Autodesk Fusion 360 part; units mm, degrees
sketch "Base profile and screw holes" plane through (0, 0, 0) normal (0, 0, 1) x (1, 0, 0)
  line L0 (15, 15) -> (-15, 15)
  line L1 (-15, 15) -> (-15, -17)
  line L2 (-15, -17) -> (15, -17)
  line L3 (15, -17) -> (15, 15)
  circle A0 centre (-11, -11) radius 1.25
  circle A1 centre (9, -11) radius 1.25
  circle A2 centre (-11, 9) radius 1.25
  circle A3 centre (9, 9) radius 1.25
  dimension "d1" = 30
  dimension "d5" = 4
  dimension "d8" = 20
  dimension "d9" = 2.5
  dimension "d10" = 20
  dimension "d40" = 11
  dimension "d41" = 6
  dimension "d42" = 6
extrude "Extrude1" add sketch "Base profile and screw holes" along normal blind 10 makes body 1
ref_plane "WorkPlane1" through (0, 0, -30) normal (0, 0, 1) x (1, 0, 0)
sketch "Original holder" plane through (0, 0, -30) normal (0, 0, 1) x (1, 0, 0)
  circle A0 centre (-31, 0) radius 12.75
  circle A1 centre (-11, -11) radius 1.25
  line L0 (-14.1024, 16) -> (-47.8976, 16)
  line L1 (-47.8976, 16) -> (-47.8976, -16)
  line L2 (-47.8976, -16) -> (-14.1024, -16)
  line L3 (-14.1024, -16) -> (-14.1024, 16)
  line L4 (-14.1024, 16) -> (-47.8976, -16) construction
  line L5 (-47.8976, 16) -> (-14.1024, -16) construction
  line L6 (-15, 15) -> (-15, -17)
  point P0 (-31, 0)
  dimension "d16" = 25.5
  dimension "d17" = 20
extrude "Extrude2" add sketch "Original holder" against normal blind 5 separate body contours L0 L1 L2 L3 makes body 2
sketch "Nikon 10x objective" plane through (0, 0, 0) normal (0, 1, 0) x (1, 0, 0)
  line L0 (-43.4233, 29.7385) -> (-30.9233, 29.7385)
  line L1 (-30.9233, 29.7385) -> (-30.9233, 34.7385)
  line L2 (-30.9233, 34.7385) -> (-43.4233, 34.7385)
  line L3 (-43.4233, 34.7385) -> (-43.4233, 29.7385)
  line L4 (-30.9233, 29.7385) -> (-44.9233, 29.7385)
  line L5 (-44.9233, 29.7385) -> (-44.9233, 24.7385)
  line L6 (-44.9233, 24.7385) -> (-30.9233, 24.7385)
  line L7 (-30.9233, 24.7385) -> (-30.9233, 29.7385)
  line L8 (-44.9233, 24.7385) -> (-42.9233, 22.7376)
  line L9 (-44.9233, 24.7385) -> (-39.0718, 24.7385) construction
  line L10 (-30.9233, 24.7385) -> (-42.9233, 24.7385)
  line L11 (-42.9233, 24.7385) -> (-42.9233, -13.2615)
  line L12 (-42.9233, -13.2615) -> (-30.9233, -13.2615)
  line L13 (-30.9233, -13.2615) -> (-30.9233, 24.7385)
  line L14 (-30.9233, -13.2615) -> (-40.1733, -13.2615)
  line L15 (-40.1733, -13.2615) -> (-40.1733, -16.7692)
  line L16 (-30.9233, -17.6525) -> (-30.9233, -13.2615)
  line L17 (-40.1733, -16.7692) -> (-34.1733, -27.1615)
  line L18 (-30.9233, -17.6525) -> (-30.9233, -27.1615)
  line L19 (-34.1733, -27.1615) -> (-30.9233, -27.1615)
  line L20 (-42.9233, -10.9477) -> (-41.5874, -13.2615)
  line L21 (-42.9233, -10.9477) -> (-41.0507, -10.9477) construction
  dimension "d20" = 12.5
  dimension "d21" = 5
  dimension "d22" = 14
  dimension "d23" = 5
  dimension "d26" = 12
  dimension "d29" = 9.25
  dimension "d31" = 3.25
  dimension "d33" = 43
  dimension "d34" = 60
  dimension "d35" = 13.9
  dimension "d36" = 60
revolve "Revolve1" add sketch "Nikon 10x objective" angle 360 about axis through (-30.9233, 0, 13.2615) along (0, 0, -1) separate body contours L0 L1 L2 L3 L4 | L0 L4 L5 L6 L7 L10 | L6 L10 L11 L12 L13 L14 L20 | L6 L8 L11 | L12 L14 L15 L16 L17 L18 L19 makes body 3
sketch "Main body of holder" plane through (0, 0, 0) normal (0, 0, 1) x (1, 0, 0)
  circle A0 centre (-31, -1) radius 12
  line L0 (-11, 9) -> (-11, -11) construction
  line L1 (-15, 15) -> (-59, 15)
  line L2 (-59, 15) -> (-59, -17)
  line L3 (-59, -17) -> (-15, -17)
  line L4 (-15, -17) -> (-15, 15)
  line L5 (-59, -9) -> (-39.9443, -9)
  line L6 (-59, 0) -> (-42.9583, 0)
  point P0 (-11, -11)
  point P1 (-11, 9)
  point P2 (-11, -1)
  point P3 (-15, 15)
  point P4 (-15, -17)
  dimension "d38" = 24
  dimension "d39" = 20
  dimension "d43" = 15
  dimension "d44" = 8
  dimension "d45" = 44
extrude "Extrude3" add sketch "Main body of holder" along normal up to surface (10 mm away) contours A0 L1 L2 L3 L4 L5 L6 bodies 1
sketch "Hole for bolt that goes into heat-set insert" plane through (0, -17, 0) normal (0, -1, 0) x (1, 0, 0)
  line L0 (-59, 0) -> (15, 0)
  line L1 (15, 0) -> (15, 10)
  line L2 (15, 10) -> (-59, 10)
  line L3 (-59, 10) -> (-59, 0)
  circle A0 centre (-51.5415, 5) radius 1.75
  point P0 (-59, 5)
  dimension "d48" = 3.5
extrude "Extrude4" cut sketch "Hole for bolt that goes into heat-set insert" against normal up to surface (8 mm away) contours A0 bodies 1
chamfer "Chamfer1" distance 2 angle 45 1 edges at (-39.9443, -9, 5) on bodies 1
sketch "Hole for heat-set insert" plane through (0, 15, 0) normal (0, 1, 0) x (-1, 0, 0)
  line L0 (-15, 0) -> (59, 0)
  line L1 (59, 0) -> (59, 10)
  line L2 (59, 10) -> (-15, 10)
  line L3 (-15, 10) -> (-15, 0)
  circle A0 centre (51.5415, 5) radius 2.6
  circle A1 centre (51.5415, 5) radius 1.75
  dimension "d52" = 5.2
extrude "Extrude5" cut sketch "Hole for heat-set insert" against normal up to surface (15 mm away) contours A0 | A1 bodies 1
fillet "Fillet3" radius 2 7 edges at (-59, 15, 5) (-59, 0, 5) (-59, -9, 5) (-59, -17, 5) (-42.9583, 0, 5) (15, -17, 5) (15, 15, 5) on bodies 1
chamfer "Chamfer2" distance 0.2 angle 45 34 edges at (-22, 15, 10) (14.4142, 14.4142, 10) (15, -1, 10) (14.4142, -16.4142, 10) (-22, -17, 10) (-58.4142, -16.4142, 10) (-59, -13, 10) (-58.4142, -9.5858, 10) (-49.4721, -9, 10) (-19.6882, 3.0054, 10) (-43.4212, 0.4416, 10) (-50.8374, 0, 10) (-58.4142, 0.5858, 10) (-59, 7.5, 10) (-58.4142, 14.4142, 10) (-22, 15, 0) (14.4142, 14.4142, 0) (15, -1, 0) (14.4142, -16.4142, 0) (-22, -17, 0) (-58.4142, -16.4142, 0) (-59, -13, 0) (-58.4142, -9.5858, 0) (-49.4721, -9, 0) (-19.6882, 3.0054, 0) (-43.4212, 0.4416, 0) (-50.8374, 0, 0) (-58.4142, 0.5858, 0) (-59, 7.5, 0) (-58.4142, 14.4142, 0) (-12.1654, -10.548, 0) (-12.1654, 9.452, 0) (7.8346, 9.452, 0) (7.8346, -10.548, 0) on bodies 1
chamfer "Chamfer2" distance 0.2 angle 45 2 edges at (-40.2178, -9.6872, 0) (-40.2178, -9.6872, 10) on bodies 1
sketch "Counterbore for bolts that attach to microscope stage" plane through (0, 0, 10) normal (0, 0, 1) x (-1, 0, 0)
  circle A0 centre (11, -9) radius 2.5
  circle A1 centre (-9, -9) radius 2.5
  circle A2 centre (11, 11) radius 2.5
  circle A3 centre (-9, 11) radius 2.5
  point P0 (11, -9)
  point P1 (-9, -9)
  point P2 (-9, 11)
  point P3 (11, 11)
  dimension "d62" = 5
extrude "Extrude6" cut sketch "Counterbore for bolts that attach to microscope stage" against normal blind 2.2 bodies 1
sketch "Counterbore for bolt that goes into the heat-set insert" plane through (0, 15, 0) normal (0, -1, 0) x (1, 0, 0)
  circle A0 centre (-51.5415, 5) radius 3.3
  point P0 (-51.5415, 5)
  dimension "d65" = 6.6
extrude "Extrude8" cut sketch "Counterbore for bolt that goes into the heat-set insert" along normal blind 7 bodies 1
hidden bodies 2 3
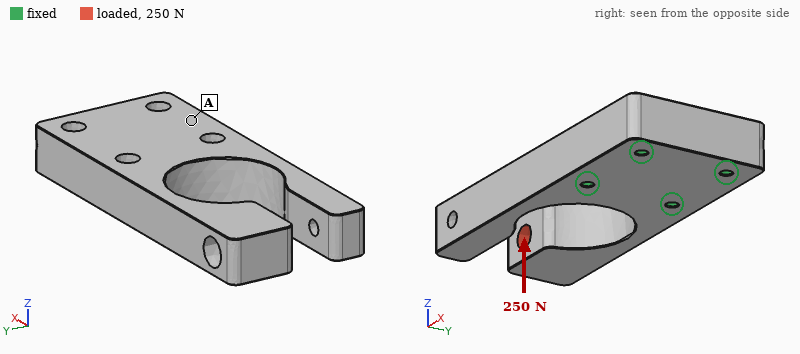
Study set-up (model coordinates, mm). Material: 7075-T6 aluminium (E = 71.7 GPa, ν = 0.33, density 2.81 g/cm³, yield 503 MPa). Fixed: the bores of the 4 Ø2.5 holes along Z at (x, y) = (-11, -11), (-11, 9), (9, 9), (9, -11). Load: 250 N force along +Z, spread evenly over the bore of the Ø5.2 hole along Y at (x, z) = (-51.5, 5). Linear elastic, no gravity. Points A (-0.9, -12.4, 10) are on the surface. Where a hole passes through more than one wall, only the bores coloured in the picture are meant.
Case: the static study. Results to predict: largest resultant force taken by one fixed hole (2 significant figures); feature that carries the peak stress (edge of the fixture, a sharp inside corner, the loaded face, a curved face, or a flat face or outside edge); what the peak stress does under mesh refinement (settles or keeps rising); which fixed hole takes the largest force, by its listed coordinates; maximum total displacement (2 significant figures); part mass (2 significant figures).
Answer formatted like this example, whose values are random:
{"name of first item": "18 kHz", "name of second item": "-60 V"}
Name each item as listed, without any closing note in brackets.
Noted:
{"largest resultant force taken by one fixed hole": "390 N", "feature that carries the peak stress": "edge of the fixture", "what the peak stress does under mesh refinement": "keeps rising", "which fixed hole takes the largest force, by its listed coordinates": "(-11, 9)", "maximum total displacement": "0.26 mm", "part mass": "47 g"}
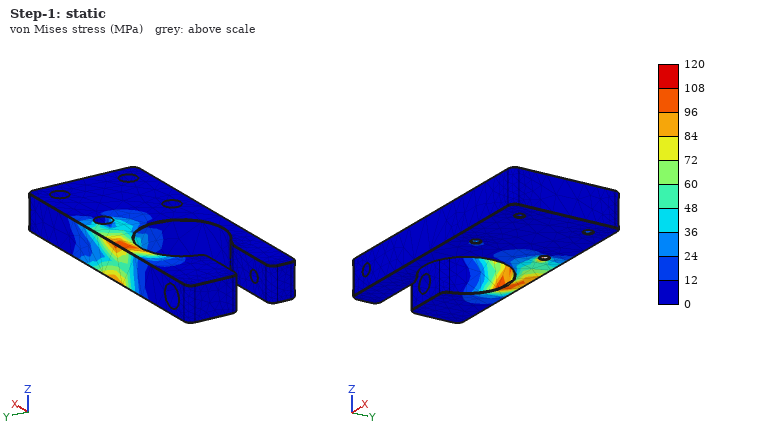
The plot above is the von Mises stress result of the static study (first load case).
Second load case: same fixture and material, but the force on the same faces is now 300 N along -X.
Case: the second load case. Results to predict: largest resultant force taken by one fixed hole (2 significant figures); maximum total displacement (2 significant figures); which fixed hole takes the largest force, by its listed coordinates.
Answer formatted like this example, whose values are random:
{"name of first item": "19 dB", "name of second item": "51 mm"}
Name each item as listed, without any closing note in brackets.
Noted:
{"largest resultant force taken by one fixed hole": "190 N", "maximum total displacement": "0.24 mm", "which fixed hole takes the largest force, by its listed coordinates": "(-11, 9)"}
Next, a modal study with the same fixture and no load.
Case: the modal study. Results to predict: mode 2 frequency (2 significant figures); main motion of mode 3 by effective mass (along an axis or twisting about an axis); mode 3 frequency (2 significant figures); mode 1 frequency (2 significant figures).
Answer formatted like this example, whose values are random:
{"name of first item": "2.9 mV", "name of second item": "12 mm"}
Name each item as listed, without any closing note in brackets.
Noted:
{"mode 2 frequency": "2100 Hz", "main motion of mode 3 by effective mass": "along Z", "mode 3 frequency": "2500 Hz", "mode 1 frequency": "1600 Hz"}
